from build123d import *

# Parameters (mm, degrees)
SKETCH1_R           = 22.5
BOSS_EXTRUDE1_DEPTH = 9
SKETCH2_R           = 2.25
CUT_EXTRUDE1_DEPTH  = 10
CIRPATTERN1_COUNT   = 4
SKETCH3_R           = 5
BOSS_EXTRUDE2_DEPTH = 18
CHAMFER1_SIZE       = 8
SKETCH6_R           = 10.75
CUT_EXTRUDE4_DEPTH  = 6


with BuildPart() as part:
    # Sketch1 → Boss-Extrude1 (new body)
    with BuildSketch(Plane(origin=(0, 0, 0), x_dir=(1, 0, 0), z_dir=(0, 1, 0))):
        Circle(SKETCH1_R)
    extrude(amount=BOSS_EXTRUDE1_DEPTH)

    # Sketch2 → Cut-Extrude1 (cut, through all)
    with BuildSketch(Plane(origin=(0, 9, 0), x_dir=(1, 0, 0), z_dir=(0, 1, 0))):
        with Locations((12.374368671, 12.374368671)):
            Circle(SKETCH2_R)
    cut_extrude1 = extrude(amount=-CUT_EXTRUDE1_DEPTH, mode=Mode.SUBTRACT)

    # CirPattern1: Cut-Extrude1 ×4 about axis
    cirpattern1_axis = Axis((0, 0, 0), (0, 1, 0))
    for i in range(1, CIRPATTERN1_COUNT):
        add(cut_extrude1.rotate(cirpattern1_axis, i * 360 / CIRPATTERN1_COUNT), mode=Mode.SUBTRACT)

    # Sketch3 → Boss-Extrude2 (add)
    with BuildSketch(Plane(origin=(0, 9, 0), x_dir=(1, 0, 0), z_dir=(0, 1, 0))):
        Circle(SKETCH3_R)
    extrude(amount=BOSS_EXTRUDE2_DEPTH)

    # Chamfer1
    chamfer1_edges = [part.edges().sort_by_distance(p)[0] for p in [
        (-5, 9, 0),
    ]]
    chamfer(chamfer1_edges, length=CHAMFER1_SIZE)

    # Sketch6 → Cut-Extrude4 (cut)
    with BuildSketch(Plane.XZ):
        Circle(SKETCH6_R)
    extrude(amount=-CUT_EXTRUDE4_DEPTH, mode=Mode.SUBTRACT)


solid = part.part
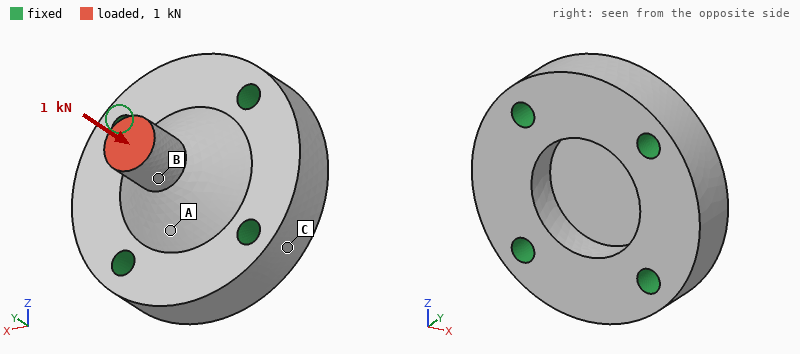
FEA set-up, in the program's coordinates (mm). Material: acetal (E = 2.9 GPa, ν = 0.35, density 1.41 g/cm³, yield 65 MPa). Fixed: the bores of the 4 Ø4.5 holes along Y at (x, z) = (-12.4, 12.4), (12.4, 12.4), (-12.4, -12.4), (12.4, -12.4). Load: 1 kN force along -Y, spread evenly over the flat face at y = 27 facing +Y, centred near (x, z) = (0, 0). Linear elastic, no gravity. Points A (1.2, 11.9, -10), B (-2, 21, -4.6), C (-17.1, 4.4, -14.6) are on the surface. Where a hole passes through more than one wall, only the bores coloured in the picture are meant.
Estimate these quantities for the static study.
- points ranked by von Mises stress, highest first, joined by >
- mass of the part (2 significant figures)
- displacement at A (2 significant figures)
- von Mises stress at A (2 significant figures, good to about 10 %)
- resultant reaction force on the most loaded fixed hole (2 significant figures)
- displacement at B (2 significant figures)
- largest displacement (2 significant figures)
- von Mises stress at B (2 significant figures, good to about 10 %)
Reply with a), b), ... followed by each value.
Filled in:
a) B > A > C
b) 20 g
c) 24 µm
d) 5.0 MPa
e) 290 N
f) 68 µm
g) 94 µm
h) 12 MPa
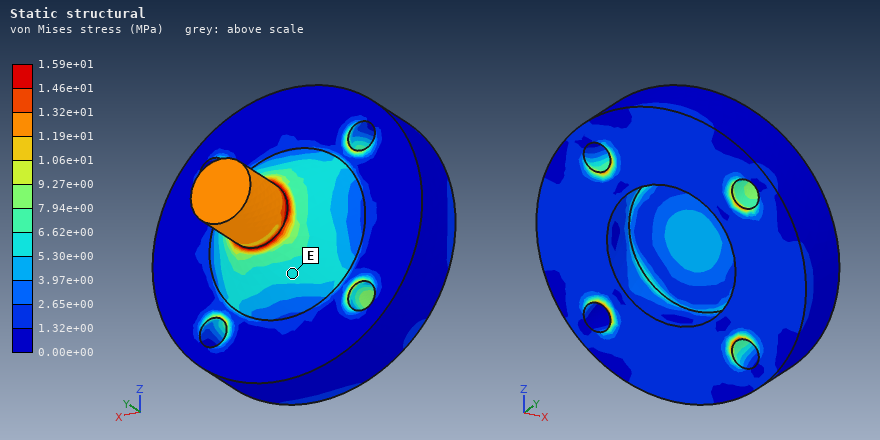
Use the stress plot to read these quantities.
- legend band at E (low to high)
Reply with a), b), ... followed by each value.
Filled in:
a) 5.30e+00 to 6.62e+00 MPa
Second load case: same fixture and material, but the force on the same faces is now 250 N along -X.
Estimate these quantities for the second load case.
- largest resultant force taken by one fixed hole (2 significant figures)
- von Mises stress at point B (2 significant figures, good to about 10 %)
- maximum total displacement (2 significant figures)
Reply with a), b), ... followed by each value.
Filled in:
a) 140 N
b) 8.5 MPa
c) 0.20 mm
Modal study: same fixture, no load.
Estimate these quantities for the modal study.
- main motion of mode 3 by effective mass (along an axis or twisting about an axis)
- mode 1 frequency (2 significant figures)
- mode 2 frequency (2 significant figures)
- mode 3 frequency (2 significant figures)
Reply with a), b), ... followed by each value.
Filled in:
a) along Y
b) 8100 Hz
c) 8100 Hz
d) 10 kHz
